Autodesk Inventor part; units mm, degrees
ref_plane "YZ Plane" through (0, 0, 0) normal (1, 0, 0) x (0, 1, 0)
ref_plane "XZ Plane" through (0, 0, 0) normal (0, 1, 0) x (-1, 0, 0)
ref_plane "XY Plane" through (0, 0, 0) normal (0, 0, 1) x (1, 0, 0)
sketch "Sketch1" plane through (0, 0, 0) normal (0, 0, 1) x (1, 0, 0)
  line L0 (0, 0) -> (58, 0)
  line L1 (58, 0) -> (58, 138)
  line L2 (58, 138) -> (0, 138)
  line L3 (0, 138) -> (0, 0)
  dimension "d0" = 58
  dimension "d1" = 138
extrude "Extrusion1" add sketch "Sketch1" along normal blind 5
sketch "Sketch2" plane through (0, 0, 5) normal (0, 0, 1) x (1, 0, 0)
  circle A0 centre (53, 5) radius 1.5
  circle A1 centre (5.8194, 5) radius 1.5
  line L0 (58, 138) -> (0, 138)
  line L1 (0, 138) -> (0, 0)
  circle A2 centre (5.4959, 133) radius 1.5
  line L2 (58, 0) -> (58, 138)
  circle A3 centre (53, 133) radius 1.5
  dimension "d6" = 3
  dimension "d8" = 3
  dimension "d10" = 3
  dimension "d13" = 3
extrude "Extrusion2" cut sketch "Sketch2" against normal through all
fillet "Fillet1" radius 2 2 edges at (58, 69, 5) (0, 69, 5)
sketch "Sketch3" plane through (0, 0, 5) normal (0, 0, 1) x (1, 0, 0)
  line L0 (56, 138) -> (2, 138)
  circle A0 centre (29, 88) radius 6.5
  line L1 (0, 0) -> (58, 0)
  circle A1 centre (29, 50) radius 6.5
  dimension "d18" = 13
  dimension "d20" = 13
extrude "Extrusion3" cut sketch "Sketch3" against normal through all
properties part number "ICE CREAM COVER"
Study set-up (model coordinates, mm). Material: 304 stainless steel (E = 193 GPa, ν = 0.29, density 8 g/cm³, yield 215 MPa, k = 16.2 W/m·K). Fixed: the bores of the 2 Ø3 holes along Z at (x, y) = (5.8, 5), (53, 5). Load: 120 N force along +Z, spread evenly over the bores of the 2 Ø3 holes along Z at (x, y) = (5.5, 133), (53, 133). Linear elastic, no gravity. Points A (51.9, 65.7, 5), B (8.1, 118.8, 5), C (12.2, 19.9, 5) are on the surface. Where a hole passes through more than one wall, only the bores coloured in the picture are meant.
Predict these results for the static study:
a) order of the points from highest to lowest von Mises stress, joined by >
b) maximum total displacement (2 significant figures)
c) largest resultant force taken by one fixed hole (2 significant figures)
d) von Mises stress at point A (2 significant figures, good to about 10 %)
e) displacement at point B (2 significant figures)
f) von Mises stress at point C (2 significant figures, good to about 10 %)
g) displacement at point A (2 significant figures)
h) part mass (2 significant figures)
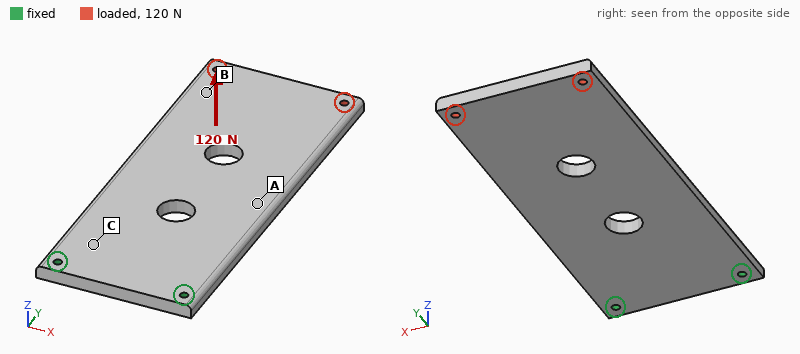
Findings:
C > A > B
0.95 mm
64 N
37 MPa
0.76 mm
57 MPa
0.27 mm
310 g
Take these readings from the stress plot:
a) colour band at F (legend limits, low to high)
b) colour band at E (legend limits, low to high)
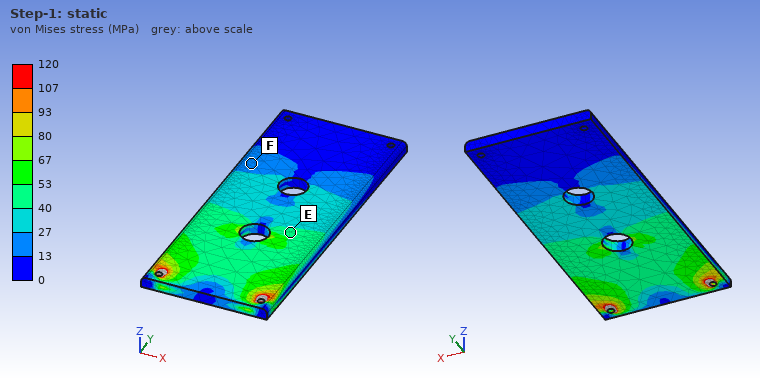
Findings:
13 to 27 MPa
40 to 53 MPa
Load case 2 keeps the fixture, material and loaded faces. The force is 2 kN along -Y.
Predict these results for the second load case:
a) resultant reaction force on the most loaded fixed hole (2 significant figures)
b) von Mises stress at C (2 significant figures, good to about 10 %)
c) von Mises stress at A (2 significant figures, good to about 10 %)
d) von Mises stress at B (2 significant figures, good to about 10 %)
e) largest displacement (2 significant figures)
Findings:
1.0 kN
8.9 MPa
8.5 MPa
11 MPa
8.2 µm
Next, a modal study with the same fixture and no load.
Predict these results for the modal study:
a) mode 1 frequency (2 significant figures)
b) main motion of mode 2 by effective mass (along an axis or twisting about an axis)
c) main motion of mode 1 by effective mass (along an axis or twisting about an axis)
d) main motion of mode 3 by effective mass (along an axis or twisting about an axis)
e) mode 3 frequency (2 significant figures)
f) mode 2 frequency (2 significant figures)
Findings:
200 Hz
twisting about Y
along Z
along Z
1300 Hz
1000 Hz
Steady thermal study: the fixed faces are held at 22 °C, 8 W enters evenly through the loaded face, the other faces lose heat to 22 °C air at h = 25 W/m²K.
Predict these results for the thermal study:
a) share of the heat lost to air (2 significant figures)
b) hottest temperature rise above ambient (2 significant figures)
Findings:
96 %
79 K
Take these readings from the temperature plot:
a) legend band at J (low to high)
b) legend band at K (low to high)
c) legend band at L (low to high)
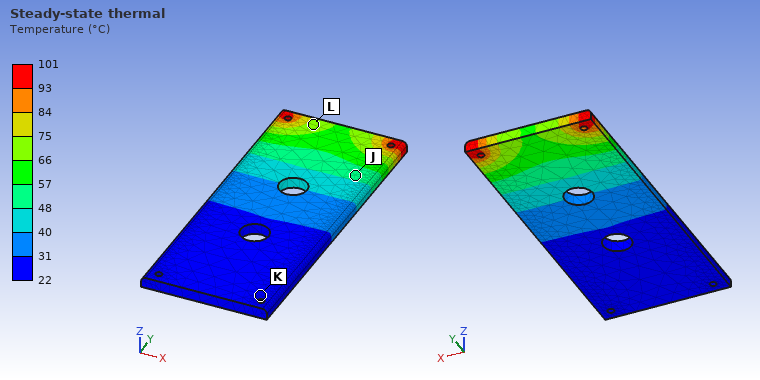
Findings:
48 to 57 °C
22 to 31 °C
66 to 75 °C
